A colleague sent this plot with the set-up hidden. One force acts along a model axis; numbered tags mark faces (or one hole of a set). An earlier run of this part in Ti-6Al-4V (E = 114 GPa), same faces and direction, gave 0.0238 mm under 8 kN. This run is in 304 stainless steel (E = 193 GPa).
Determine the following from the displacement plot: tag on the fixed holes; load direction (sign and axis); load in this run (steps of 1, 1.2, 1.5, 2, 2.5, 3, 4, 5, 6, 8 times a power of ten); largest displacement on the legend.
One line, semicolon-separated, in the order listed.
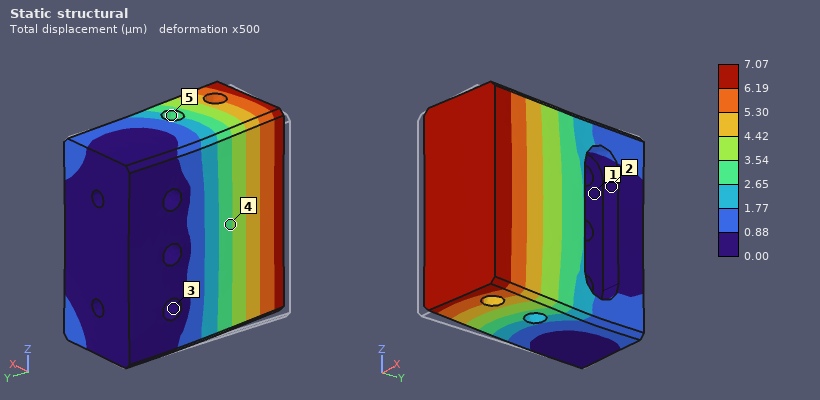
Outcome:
3; +X; 4 kN; 7.07 µm
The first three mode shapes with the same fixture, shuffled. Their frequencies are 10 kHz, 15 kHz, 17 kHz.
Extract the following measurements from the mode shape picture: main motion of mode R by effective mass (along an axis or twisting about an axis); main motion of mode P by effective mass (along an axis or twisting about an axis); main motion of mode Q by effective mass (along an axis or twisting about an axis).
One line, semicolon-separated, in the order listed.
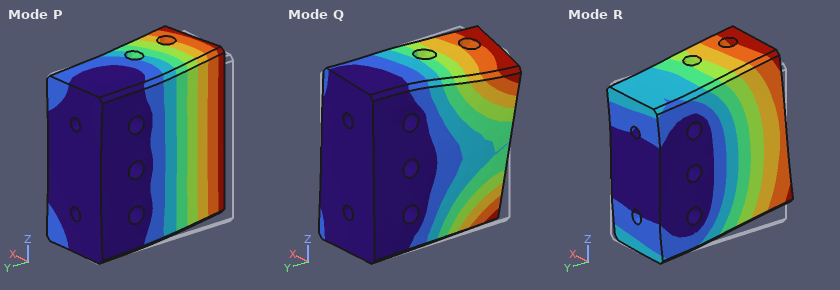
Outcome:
along Z; along X; twisting about Y
